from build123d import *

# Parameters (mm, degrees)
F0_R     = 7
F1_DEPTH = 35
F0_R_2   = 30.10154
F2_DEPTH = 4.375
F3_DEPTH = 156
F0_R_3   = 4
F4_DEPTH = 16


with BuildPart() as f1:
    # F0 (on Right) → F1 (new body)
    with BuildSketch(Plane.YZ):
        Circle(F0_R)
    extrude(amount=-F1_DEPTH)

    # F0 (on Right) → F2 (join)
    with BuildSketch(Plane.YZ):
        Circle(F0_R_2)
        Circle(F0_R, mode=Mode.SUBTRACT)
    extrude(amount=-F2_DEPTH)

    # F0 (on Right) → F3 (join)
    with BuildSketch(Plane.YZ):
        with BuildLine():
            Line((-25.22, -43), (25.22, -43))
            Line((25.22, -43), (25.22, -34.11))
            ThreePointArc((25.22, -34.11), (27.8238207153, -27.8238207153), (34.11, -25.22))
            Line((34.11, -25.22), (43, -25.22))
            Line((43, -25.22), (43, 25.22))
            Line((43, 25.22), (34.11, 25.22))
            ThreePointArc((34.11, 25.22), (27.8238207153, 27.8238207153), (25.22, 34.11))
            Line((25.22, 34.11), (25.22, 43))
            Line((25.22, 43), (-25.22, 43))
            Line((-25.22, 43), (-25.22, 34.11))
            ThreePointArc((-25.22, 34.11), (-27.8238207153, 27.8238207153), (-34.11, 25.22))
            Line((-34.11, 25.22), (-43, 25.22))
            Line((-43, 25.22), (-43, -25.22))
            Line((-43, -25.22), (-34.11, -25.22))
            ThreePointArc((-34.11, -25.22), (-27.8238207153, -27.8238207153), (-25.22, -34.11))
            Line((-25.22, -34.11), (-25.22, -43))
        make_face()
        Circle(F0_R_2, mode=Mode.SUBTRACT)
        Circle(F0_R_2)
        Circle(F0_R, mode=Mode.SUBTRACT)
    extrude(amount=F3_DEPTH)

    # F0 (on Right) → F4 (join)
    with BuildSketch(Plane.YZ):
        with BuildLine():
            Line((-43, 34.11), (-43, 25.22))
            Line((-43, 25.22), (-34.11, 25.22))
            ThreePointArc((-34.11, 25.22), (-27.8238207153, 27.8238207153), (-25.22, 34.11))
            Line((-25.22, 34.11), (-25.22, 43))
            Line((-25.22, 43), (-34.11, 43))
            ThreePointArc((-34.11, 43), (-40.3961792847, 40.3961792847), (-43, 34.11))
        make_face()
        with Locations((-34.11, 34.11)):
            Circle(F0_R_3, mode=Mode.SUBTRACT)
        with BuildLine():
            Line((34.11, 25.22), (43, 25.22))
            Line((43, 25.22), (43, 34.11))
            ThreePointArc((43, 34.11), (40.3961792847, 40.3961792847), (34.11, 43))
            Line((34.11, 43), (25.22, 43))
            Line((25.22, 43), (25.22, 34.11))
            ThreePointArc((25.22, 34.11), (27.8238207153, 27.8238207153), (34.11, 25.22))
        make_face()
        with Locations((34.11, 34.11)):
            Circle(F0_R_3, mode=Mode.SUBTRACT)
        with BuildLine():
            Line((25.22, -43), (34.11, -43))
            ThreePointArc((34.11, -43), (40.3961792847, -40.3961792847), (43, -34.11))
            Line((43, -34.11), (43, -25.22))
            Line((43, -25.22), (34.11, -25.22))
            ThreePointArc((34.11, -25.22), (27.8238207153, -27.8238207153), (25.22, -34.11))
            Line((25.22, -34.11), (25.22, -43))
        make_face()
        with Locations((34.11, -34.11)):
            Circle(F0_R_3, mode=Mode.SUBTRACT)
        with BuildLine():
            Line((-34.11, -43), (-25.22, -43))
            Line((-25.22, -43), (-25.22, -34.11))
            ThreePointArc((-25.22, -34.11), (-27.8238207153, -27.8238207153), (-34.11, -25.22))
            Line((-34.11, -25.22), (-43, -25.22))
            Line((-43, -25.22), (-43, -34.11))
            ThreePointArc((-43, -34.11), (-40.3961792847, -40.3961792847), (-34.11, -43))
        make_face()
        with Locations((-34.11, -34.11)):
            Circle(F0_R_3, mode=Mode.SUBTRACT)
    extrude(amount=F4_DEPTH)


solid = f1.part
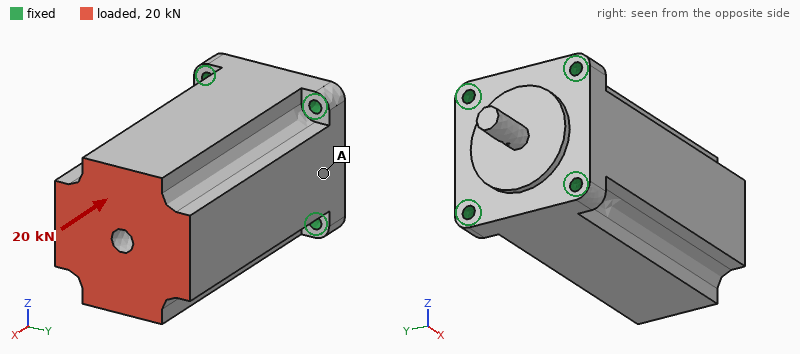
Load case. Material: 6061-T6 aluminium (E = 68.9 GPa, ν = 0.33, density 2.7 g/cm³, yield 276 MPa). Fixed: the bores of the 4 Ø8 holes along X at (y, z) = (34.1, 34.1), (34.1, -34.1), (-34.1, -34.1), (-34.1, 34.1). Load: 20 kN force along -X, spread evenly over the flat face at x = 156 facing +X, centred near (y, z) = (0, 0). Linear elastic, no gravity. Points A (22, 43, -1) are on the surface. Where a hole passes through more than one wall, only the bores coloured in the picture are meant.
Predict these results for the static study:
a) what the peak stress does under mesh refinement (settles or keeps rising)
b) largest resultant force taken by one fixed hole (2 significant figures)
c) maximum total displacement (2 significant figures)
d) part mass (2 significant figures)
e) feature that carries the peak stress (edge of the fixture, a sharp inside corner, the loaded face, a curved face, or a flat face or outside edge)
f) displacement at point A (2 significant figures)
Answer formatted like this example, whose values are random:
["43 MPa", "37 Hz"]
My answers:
["keeps rising", "5.2 kN", "13 µm", "2.6 kg", "edge of the fixture", "7.3 µm"]
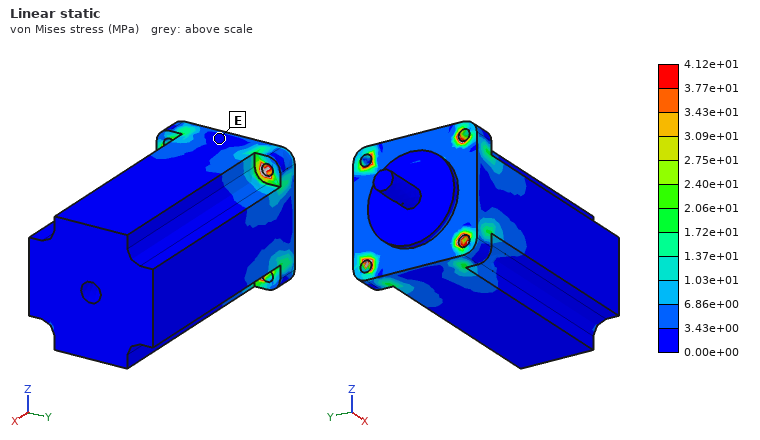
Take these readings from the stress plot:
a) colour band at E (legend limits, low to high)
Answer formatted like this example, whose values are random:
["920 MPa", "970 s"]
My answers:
["0.00e+00 to 3.43e+00 MPa"]
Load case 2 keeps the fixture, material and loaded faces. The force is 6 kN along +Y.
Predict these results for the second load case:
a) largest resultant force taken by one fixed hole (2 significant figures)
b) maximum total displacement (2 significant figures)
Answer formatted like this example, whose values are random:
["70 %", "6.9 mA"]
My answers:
["7.0 kN", "77 µm"]
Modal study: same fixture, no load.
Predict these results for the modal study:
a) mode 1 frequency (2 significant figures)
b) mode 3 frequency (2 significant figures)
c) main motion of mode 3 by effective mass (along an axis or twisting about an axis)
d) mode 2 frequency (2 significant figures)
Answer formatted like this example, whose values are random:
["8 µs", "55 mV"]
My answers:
["1600 Hz", "4700 Hz", "twisting about X", "1600 Hz"]
